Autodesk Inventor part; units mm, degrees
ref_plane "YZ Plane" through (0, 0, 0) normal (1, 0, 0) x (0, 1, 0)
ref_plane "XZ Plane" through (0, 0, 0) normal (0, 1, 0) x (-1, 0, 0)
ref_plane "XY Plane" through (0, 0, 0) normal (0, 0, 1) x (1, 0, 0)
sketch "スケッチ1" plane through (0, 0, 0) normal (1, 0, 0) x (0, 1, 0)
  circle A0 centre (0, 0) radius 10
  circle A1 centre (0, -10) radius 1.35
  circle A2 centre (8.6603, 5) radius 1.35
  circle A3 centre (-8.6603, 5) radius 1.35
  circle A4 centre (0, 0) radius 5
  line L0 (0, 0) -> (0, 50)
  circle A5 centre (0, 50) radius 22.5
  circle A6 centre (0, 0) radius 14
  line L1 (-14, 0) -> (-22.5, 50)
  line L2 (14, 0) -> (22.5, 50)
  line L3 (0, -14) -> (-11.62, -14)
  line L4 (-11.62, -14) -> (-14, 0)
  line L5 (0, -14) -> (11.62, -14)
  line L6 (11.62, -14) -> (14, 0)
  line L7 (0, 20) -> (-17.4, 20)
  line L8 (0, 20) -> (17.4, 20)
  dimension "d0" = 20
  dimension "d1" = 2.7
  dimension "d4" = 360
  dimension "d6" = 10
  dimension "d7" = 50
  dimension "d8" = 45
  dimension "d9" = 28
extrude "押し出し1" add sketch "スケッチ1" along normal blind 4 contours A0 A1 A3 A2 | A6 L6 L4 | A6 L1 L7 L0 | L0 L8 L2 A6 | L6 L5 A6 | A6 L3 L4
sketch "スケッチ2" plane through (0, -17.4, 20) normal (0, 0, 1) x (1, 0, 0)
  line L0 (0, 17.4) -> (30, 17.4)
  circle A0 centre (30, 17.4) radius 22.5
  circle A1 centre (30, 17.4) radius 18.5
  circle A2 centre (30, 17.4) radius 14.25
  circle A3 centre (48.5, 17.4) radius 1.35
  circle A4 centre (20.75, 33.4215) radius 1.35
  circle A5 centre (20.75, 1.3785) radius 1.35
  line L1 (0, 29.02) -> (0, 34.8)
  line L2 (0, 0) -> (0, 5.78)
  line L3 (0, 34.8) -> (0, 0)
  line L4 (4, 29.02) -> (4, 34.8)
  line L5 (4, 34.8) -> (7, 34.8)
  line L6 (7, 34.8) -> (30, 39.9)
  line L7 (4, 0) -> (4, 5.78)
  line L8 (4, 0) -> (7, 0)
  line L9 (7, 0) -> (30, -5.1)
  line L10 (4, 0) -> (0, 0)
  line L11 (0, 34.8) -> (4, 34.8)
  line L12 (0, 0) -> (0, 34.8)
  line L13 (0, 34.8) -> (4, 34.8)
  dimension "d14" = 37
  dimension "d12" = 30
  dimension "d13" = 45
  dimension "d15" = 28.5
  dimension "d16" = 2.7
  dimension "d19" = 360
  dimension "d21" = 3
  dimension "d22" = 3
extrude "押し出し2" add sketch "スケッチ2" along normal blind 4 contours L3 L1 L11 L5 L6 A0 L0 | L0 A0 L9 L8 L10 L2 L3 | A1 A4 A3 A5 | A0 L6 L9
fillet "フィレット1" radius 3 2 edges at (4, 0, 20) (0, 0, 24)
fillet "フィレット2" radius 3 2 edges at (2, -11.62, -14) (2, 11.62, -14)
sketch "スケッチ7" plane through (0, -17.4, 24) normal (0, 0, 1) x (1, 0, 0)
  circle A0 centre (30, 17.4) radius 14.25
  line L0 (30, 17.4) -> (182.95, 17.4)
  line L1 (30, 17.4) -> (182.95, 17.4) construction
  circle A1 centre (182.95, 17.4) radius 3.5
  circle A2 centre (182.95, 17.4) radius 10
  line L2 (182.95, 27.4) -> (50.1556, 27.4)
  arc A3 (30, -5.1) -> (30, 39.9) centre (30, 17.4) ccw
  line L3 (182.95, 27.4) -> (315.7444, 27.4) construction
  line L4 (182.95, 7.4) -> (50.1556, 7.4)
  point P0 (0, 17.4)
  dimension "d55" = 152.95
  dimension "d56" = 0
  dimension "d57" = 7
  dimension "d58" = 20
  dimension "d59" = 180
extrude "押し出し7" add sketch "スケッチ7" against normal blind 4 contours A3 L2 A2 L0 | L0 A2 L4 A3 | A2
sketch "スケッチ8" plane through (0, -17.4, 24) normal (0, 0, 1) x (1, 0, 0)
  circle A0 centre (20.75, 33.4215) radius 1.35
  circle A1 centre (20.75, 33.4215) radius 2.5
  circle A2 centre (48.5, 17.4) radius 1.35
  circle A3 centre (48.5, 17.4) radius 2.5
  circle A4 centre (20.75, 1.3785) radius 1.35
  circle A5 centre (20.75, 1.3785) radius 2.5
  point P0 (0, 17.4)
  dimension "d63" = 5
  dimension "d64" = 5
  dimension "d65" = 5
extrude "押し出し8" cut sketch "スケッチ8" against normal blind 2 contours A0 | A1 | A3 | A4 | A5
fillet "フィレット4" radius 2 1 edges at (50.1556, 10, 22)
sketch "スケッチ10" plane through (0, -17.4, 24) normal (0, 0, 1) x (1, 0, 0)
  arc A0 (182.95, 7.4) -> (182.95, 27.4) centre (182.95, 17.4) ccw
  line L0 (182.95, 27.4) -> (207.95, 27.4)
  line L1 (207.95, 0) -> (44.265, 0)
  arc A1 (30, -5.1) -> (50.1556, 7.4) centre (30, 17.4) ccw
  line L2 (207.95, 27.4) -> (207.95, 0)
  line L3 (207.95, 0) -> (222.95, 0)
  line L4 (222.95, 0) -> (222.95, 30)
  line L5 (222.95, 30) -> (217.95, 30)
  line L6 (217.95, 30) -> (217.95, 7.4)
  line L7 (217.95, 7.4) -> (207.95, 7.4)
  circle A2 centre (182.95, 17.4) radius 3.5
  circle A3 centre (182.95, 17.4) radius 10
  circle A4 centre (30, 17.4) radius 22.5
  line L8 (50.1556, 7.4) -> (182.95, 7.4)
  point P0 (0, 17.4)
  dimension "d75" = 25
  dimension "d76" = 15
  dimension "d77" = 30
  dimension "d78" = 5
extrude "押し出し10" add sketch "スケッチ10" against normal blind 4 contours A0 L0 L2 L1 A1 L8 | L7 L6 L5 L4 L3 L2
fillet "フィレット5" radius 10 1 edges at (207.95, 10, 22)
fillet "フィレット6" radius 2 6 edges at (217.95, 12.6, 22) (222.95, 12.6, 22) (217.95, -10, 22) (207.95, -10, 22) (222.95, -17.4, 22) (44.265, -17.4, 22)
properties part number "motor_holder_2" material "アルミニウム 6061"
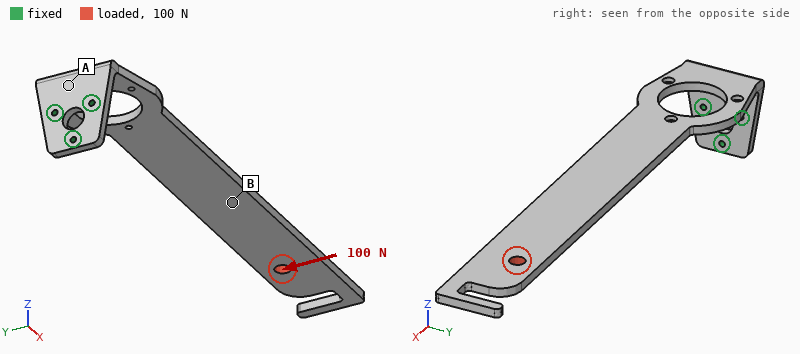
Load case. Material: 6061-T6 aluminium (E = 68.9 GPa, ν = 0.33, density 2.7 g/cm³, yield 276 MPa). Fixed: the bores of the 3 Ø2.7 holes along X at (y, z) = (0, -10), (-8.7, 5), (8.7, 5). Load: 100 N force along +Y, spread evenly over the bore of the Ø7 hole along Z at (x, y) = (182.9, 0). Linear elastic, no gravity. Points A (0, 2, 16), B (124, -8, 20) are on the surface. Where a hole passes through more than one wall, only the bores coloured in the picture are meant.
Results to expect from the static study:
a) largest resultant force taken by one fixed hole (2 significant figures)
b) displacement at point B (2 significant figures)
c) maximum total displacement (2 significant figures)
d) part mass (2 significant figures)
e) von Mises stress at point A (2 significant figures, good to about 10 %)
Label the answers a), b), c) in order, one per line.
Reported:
a) 870 N
b) 1.1 mm
c) 2.2 mm
d) 72 g
e) 96 MPa
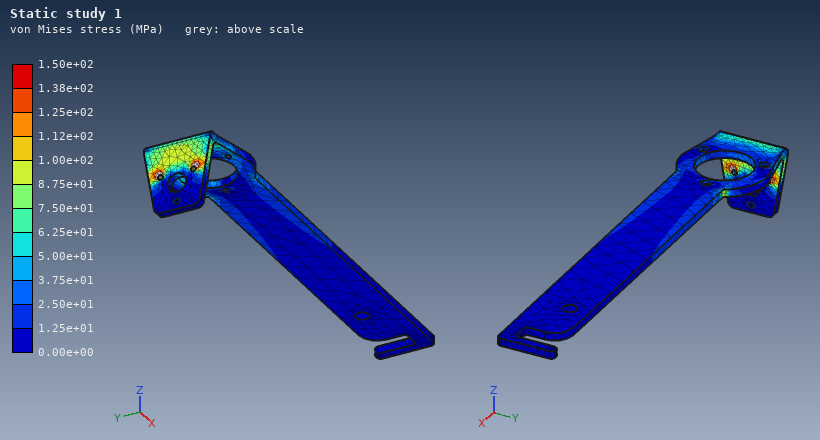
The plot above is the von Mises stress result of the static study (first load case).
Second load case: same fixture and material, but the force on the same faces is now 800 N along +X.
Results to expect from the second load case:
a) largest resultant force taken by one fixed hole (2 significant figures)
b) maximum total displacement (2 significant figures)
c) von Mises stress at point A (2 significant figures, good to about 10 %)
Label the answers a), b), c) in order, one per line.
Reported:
a) 450 N
b) 2.4 mm
c) 47 MPa
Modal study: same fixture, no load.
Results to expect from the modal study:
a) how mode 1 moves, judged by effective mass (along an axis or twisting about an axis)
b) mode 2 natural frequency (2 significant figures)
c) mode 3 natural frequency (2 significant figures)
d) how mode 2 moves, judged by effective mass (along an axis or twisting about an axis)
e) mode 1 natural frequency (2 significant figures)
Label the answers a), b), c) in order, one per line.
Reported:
a) along Z
b) 230 Hz
c) 400 Hz
d) along Y
e) 57 Hz
